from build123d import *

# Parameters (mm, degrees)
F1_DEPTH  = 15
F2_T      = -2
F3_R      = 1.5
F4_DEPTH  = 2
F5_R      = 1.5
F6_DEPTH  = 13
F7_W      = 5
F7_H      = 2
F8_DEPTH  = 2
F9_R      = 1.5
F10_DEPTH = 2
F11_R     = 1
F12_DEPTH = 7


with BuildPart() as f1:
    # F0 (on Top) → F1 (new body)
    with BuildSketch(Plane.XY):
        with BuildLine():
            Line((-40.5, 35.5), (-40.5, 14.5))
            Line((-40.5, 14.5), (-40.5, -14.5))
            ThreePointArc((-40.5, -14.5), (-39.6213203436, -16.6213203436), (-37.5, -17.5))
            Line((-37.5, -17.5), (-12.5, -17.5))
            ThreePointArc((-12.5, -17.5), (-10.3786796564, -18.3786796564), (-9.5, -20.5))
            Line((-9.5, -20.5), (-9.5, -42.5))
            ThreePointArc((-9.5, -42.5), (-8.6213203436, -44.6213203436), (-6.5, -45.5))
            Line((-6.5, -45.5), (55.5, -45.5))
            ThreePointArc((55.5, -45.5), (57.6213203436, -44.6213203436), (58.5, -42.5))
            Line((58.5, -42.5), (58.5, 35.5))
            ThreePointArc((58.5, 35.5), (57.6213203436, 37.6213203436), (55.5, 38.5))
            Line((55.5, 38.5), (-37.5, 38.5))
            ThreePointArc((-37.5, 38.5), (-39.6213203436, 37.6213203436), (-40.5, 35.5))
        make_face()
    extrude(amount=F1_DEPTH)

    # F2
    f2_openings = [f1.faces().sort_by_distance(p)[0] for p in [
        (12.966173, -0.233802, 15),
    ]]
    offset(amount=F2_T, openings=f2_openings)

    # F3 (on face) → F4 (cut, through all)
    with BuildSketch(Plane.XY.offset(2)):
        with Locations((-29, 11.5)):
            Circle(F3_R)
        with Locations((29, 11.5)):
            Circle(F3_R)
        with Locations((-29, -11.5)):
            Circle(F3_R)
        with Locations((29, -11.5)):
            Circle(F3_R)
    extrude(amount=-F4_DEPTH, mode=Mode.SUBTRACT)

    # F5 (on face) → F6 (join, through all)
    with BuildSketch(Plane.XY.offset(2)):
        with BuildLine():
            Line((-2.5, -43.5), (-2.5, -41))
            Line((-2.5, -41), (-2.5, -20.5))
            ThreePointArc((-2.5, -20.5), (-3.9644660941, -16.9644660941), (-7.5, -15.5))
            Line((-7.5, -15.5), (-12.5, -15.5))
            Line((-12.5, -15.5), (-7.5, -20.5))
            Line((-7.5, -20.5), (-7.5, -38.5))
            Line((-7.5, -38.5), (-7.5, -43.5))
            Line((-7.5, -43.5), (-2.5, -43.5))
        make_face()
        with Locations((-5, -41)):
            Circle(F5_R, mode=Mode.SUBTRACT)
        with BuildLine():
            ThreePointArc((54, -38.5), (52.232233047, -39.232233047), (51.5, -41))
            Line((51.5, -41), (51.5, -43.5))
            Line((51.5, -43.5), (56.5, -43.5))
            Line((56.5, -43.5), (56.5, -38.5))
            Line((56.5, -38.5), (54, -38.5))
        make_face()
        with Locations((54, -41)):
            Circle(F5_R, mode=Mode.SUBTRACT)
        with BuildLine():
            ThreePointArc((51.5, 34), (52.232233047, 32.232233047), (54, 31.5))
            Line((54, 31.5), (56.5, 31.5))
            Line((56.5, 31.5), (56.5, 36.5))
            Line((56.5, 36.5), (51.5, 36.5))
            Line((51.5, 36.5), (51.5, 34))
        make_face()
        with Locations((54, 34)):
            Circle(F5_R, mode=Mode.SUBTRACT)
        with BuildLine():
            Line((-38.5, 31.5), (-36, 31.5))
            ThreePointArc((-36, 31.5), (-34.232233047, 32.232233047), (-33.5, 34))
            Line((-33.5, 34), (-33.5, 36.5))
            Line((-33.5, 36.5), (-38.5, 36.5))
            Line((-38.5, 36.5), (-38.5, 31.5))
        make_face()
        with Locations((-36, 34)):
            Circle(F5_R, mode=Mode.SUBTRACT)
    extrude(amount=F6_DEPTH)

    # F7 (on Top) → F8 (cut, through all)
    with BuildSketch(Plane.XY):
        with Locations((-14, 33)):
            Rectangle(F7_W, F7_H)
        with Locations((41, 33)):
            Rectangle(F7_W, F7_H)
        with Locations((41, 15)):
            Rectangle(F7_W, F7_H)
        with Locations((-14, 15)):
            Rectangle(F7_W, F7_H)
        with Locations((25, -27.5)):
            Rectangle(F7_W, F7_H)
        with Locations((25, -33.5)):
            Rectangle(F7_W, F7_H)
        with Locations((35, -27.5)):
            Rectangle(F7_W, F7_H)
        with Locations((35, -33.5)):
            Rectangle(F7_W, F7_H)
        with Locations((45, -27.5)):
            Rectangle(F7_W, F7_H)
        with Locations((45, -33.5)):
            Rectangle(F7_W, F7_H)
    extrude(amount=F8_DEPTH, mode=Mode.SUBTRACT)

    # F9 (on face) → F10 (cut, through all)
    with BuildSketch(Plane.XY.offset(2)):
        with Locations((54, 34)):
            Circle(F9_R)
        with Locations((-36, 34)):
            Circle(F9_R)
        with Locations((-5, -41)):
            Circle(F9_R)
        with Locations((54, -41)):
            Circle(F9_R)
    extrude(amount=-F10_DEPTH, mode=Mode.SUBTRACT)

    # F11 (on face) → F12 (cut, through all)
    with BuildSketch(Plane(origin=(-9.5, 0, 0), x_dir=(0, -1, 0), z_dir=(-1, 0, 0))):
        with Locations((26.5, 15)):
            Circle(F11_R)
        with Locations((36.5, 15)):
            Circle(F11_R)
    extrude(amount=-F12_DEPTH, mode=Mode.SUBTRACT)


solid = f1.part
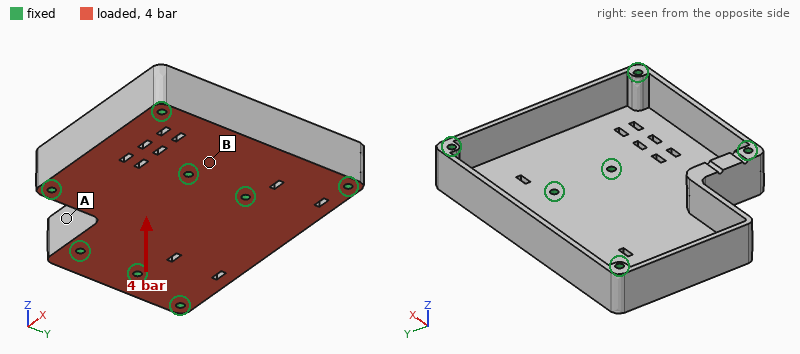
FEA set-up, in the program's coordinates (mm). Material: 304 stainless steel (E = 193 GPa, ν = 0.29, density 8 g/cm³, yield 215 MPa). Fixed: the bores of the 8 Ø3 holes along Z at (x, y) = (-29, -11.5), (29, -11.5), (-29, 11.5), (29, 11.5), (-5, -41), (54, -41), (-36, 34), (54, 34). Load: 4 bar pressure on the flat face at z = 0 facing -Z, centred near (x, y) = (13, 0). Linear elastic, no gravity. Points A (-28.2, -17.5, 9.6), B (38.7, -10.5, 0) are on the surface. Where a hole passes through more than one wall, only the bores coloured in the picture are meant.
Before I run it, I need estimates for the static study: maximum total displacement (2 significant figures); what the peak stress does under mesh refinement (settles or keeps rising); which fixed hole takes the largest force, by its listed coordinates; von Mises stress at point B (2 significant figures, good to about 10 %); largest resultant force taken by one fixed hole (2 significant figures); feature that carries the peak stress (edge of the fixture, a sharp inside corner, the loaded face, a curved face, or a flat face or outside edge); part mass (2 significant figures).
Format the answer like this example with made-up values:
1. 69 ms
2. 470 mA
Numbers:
1. 55 µm
2. keeps rising
3. (-5, -41)
4. 18 MPa
5. 660 N
6. edge of the fixture
7. 210 g
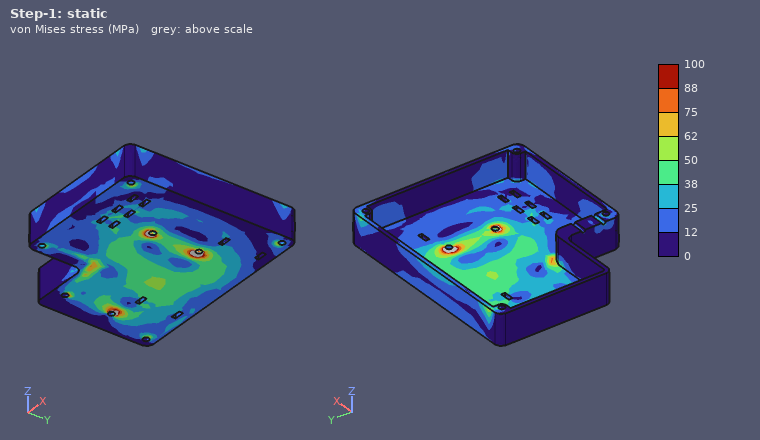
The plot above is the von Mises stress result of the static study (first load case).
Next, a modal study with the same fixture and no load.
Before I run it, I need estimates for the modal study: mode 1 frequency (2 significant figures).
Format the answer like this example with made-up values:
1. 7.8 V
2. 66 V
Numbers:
1. 4000 Hz
